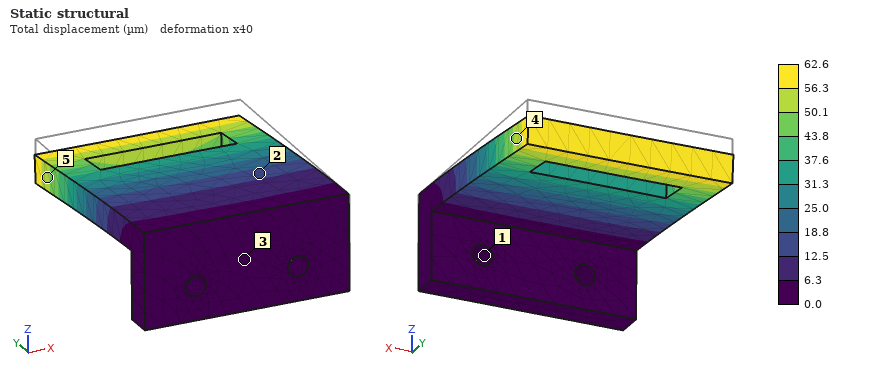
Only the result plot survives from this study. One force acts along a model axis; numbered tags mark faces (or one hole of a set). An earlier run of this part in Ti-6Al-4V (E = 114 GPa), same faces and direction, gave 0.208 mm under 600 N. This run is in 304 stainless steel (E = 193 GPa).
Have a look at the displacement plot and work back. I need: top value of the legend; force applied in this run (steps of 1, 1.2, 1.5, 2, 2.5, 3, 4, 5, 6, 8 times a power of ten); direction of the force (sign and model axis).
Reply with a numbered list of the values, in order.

1. 62.6 µm
2. 300 N
3. -Z
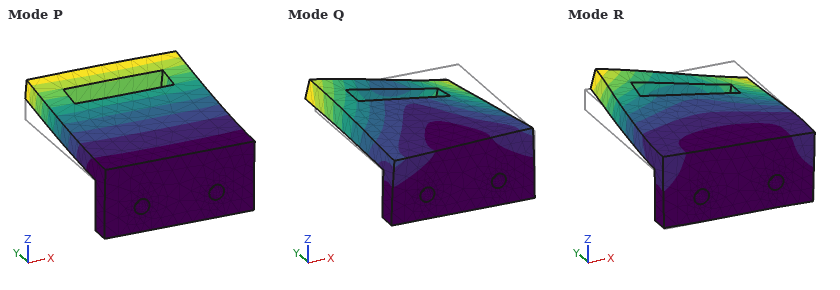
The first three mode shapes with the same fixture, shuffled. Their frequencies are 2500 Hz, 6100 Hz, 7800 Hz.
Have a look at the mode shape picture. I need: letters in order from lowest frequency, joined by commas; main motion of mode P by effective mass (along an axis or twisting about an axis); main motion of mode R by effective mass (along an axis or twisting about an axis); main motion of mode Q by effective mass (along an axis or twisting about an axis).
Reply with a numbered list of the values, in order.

1. P, Q, R
2. along Z
3. along X
4. along X
